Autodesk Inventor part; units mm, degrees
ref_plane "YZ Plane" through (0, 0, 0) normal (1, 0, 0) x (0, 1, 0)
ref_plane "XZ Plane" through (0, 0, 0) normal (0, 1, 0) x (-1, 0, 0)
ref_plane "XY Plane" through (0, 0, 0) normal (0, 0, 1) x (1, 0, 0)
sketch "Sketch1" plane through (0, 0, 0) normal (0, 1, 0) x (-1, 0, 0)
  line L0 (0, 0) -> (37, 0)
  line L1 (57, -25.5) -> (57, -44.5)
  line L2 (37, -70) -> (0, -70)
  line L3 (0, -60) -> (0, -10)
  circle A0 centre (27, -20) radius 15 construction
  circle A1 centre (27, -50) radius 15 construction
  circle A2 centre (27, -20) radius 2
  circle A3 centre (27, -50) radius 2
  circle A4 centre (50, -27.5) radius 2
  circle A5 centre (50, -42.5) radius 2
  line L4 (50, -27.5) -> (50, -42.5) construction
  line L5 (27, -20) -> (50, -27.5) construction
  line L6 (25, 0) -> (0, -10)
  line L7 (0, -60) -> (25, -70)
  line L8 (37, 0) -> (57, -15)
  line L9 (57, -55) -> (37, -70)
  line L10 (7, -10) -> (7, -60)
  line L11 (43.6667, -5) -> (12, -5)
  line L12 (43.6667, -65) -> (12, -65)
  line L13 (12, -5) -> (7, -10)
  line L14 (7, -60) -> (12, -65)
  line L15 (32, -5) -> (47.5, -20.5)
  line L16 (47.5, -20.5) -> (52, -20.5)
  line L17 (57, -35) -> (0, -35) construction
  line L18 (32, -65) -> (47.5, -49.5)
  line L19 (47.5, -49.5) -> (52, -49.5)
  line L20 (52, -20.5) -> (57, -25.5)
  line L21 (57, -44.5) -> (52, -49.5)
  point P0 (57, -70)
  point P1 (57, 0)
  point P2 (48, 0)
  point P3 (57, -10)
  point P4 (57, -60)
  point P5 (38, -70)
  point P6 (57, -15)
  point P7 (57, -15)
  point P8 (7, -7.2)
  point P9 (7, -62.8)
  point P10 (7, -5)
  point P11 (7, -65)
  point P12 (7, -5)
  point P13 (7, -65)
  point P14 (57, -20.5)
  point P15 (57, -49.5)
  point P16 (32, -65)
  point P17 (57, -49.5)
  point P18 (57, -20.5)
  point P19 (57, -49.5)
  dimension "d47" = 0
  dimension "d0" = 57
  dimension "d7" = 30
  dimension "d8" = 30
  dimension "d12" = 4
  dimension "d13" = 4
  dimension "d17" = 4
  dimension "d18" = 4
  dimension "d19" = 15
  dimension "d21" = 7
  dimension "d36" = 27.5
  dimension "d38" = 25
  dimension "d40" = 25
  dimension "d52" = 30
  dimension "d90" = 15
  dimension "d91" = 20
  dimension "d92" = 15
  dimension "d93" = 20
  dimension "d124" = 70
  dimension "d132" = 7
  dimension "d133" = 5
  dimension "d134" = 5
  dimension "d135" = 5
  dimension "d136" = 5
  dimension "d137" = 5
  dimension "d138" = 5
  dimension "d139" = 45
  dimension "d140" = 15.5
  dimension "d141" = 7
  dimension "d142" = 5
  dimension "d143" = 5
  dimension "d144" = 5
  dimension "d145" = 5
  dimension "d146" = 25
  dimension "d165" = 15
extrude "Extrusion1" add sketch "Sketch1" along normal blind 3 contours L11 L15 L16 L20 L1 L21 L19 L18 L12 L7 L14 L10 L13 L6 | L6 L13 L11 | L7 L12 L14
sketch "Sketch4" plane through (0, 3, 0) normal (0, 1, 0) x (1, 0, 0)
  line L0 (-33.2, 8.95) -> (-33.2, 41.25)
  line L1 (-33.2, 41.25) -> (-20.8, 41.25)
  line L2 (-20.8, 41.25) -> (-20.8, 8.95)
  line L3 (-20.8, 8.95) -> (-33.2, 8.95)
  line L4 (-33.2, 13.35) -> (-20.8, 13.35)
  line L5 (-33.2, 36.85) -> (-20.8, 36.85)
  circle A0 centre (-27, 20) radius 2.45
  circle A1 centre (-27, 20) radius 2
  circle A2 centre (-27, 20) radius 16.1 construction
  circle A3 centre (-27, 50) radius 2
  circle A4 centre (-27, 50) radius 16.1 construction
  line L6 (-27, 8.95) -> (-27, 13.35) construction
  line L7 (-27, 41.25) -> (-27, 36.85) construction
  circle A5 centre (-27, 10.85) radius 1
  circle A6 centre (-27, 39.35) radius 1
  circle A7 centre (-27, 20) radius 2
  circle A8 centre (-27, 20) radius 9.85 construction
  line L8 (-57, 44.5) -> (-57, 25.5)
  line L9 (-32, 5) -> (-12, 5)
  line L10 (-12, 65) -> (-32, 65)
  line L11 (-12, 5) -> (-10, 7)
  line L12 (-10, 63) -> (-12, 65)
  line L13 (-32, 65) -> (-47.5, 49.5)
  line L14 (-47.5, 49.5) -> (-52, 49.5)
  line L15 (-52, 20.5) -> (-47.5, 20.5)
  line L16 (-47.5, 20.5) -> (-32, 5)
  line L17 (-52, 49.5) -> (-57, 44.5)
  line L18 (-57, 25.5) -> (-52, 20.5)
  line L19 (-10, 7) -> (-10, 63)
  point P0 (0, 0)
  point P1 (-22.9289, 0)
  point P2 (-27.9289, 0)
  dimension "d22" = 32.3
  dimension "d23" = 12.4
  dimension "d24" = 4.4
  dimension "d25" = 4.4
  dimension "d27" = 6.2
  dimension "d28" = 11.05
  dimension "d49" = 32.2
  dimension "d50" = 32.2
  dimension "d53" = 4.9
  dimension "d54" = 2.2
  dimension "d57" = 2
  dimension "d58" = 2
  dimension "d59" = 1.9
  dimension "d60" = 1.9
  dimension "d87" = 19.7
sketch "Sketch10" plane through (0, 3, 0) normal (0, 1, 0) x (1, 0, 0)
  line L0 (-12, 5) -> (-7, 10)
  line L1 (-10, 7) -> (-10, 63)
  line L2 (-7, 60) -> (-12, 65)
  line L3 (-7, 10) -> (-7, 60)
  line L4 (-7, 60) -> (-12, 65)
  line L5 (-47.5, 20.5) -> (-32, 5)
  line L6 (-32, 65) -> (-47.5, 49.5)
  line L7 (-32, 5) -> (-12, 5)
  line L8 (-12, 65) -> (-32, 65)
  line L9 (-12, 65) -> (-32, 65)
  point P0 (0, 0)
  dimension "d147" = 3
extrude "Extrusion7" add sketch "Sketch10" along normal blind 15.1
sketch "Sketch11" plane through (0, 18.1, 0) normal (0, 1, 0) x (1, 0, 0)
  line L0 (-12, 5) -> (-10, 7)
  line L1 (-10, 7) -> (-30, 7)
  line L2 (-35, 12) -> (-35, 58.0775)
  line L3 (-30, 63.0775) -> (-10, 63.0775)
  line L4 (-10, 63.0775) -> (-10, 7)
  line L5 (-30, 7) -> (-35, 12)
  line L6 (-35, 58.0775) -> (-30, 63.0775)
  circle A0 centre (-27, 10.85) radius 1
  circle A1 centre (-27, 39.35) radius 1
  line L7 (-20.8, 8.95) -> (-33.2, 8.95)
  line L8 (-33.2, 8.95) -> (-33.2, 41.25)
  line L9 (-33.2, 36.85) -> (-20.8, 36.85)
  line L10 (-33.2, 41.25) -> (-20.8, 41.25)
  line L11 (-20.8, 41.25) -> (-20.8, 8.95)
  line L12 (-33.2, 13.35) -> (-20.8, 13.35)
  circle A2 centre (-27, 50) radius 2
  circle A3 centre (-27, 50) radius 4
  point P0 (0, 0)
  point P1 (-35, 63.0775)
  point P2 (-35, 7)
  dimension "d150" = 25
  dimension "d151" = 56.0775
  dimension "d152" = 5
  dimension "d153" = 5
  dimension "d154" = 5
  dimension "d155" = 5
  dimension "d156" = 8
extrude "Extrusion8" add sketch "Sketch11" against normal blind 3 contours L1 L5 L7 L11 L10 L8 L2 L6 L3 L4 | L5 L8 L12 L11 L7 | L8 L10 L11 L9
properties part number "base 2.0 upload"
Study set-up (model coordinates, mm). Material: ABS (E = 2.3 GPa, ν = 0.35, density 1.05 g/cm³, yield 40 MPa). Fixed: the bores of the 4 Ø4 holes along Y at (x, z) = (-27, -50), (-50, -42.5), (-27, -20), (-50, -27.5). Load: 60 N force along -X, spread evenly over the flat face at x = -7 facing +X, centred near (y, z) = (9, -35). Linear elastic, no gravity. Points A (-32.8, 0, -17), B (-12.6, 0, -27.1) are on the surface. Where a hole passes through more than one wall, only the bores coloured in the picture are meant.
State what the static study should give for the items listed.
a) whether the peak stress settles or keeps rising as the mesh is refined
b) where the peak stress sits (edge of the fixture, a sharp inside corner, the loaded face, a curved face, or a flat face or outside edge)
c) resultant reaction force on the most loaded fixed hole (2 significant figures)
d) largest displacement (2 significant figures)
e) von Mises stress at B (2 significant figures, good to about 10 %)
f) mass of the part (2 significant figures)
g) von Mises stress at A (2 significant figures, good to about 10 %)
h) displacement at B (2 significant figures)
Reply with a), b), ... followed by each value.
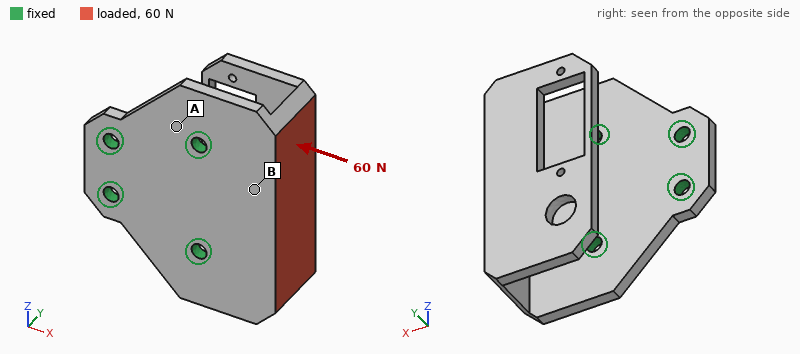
a) keeps rising
b) edge of the fixture
c) 25 N
d) 0.80 mm
e) 4.4 MPa
f) 13 g
g) 1.1 MPa
h) 0.16 mm
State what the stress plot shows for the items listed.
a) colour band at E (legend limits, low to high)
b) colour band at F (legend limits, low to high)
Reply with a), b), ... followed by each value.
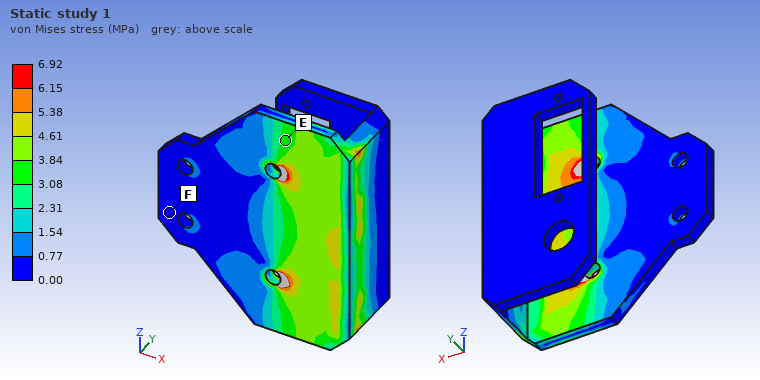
a) 3.08 to 3.84 MPa
b) 0.00 to 0.77 MPa
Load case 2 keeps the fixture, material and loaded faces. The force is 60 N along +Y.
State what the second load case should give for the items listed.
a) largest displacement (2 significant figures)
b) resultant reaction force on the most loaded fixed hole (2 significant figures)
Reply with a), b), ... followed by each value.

a) 0.89 mm
b) 36 N
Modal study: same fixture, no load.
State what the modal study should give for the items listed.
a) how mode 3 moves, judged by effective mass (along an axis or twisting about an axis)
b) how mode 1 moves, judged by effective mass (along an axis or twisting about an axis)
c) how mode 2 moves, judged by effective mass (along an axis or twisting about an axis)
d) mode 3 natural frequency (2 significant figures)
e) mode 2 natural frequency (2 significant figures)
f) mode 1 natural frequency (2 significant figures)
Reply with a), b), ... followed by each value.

a) along Y
b) along X
c) along Z
d) 790 Hz
e) 690 Hz
f) 470 Hz
